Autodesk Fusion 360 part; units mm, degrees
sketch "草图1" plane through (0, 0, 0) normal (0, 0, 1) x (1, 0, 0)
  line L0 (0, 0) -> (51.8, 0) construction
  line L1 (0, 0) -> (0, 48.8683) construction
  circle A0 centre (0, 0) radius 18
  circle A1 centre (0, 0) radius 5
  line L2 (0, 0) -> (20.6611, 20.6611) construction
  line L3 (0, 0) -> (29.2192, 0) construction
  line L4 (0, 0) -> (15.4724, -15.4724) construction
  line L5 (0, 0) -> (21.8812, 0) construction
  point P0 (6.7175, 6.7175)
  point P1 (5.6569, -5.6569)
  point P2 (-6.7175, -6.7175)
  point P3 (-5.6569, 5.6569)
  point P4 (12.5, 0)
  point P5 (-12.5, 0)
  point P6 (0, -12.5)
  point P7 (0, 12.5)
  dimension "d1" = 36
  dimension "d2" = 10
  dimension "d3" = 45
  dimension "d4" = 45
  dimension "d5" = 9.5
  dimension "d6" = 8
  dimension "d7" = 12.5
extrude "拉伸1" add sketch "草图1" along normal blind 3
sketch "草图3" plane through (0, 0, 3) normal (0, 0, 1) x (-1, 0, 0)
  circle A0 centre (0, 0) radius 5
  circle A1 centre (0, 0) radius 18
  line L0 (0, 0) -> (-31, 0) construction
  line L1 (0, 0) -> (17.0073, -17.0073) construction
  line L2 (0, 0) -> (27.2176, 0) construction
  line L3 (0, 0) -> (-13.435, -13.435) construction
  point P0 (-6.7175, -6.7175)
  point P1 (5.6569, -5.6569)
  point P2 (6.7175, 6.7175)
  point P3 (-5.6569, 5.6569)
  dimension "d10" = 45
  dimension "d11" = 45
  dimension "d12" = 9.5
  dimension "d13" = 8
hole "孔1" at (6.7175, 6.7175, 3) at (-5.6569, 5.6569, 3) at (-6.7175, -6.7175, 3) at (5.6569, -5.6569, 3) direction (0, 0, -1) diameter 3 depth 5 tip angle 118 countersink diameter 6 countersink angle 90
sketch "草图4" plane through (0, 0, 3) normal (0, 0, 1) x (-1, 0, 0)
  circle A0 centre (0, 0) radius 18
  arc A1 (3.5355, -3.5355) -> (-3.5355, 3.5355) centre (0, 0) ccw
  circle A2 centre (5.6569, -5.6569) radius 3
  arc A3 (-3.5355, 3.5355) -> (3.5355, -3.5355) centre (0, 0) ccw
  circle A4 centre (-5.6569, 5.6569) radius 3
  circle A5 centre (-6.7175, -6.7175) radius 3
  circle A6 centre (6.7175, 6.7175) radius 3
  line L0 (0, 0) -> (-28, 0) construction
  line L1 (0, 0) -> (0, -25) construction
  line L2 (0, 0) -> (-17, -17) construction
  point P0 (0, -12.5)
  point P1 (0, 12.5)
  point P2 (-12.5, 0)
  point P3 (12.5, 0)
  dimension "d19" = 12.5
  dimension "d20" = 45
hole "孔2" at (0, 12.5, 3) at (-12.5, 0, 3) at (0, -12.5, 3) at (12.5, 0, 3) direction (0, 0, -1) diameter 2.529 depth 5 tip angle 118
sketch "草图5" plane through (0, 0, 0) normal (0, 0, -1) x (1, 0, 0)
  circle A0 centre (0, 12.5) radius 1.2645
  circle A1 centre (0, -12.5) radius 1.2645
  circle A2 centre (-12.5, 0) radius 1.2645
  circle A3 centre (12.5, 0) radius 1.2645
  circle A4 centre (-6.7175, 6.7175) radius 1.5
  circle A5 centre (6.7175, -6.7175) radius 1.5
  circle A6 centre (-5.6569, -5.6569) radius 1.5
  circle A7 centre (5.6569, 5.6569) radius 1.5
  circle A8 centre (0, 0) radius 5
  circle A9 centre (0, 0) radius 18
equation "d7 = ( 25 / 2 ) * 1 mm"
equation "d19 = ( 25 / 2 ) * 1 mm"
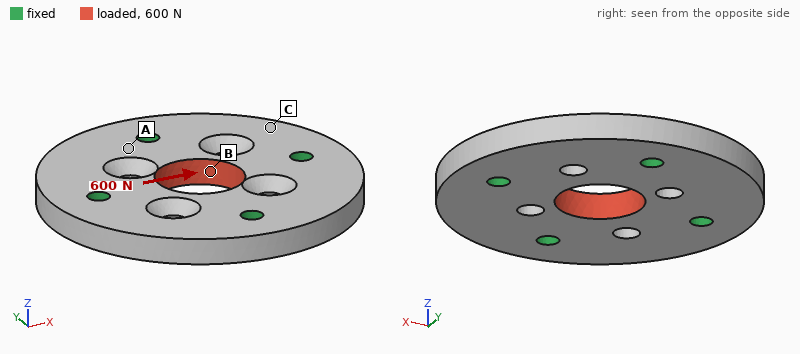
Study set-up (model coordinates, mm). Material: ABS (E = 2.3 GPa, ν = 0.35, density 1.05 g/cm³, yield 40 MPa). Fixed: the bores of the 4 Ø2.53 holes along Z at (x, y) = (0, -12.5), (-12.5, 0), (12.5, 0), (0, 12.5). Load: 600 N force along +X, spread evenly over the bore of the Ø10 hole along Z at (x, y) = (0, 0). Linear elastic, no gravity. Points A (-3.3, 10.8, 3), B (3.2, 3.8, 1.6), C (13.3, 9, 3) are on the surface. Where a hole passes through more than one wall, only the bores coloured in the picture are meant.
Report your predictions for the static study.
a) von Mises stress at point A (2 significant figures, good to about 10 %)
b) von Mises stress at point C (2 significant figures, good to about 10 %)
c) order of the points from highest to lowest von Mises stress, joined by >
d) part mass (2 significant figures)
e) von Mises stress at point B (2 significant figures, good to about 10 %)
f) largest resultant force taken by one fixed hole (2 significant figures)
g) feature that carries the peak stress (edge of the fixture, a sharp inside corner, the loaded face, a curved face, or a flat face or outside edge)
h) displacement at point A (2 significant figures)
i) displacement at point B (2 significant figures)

4.0 MPa
1.8 MPa
B > A > C
2.7 g
11 MPa
190 N
a curved face
10 µm
38 µm
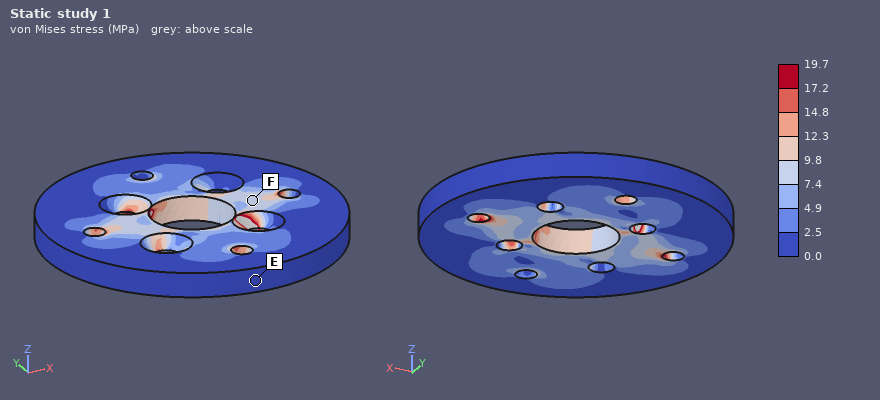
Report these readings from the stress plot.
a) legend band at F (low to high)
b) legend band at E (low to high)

7.4 to 9.8 MPa
0.0 to 2.5 MPa
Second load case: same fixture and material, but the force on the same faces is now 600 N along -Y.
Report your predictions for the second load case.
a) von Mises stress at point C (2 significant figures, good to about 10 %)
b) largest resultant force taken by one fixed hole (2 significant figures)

2.0 MPa
190 N
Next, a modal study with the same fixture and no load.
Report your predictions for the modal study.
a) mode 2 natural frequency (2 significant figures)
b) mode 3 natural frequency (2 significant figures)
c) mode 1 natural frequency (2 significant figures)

7800 Hz
7800 Hz
7300 Hz
